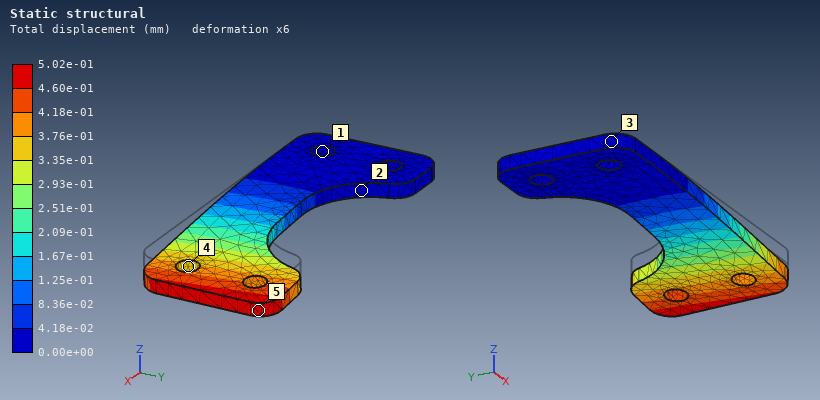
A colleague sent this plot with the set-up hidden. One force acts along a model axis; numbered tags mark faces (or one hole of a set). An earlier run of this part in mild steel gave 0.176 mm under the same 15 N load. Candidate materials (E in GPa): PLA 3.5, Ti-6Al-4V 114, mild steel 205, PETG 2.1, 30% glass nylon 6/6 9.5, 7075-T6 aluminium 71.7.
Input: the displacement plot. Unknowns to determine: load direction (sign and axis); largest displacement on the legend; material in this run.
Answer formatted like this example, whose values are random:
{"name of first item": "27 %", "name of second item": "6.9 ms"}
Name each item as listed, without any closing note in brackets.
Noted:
{"load direction": "-Z", "largest displacement on the legend": "5.02e-01 mm", "material in this run": "7075-T6 aluminium"}
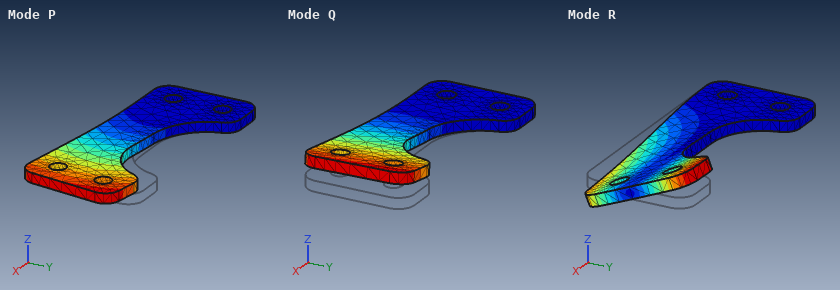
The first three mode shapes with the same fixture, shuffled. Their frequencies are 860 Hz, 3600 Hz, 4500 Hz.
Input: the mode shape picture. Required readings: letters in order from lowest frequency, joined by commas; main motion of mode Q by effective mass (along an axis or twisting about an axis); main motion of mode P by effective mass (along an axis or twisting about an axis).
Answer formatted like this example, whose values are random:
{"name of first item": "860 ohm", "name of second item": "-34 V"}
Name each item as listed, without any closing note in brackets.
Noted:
{"letters in order from lowest frequency, joined by commas": "Q, R, P", "main motion of mode Q by effective mass": "along Z", "main motion of mode P by effective mass": "along Y"}
